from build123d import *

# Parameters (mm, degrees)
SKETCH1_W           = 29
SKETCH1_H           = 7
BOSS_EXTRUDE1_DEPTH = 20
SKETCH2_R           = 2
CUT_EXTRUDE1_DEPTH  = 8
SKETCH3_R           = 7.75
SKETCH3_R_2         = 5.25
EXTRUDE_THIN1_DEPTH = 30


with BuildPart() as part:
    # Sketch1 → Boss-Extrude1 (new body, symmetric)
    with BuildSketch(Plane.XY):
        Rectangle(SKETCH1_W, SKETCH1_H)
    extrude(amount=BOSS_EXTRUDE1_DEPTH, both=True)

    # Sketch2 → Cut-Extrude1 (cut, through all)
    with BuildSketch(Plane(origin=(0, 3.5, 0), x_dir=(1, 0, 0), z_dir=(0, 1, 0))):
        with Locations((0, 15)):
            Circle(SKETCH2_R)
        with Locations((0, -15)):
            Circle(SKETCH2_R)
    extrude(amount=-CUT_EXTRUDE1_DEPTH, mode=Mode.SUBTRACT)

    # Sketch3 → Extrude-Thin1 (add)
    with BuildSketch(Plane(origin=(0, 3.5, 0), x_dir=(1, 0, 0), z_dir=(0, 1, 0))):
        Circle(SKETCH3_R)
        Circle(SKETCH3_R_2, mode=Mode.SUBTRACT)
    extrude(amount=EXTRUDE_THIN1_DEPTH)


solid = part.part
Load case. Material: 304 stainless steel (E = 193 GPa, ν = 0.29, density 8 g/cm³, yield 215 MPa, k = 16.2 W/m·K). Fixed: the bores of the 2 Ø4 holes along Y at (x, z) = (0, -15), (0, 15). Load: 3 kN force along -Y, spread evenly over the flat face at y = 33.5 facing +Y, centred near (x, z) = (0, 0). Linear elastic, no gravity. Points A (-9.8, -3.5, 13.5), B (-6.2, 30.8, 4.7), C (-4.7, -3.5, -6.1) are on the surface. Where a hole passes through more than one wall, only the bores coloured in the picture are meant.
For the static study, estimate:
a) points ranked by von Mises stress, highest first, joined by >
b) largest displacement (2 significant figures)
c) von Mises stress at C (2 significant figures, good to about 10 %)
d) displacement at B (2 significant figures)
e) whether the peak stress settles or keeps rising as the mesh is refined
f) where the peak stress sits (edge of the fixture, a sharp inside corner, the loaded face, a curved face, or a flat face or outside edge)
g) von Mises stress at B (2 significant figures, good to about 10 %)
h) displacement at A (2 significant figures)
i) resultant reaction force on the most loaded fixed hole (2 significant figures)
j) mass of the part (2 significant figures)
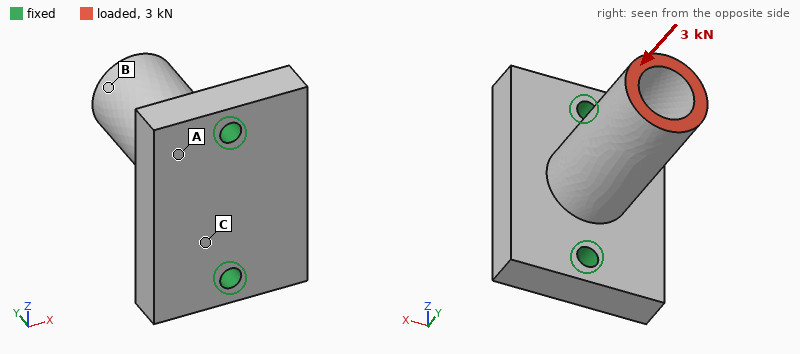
B > C > A
8.4 µm
19 MPa
8.0 µm
keeps rising
edge of the fixture
29 MPa
1.8 µm
1.5 kN
88 g
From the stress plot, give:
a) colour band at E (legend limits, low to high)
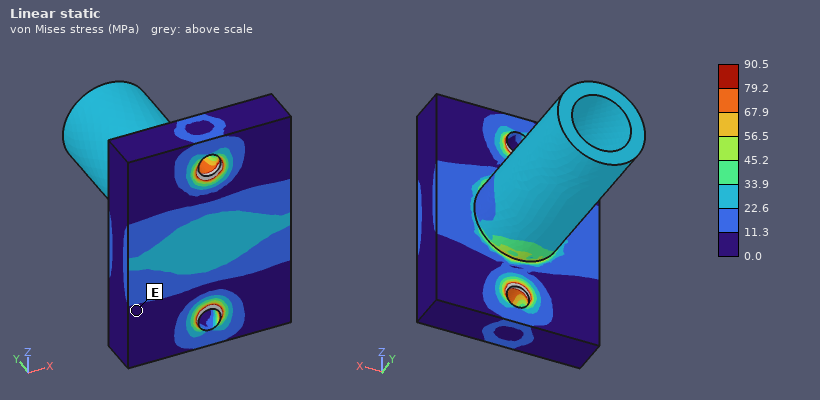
0.0 to 11.3 MPa
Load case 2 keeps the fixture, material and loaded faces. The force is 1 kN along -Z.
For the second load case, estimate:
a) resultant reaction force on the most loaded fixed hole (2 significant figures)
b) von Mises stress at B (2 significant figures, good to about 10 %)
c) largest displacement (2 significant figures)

1.4 kN
23 MPa
42 µm
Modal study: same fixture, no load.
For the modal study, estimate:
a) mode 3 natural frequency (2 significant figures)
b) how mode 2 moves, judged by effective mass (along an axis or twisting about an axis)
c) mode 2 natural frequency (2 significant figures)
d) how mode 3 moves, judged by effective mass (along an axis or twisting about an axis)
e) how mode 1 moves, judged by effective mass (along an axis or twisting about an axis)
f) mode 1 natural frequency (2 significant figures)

17 kHz
along Z
9100 Hz
along Y
along X
6400 Hz
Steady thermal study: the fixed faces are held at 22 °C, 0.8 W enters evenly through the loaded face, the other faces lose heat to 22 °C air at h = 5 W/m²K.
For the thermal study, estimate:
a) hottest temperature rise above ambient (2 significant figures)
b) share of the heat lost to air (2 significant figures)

15 K
15 %
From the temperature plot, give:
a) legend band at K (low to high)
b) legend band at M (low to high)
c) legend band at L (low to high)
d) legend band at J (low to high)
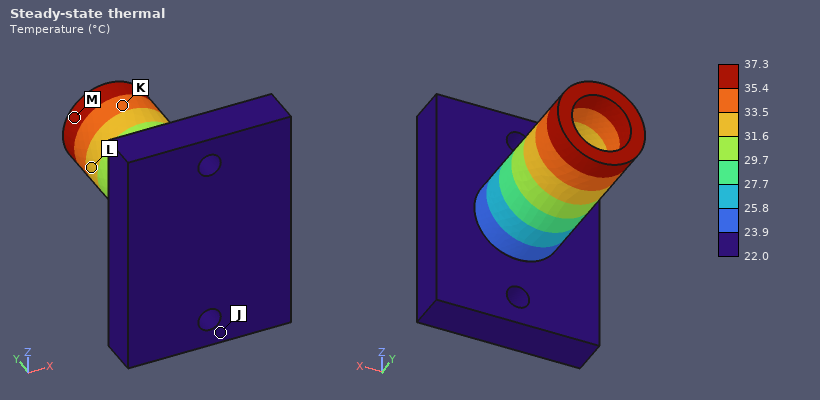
33.5 to 35.4 °C
35.4 to 37.3 °C
31.6 to 33.5 °C
22.0 to 23.9 °C
